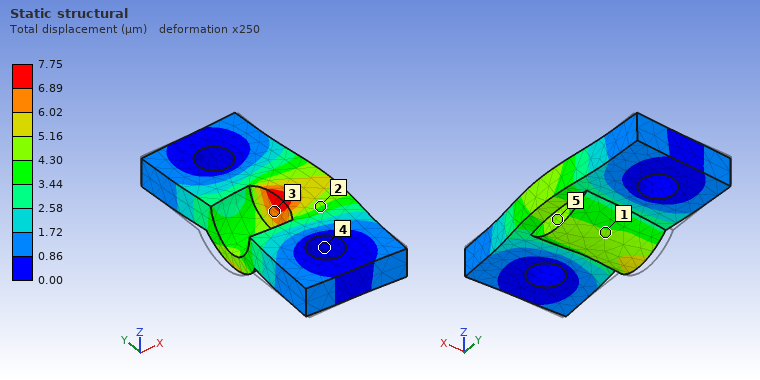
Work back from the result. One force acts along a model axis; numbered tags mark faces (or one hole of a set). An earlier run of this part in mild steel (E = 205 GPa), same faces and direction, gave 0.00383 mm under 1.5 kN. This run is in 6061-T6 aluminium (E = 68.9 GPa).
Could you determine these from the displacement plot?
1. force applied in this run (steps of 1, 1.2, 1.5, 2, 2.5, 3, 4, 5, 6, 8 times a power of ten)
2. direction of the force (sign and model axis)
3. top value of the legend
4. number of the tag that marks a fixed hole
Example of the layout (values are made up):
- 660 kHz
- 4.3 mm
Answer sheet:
- 1 kN
- +X
- 7.75 µm
- 4
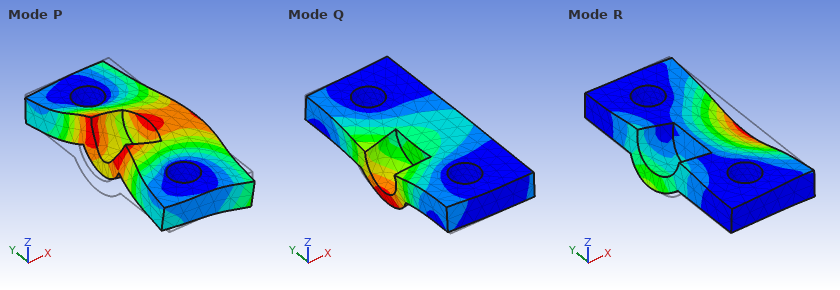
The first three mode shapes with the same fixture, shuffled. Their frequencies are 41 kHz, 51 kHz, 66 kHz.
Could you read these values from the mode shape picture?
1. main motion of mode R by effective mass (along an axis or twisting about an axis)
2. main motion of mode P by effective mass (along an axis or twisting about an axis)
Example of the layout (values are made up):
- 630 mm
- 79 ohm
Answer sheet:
- along Z
- along X
